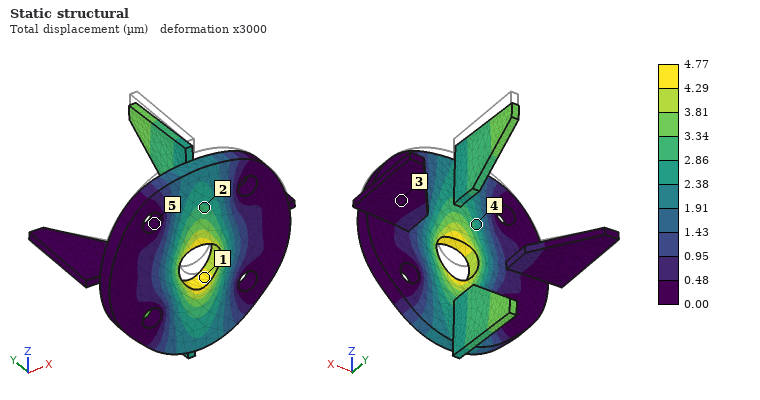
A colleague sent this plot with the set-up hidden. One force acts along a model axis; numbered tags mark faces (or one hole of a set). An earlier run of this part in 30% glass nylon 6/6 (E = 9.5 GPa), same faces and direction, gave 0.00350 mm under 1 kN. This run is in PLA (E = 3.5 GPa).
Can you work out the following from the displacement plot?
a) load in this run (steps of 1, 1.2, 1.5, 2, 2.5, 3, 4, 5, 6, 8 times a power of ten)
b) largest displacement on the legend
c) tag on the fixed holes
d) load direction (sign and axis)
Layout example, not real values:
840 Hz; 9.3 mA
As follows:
500 N; 4.77 µm; 5; -Z
